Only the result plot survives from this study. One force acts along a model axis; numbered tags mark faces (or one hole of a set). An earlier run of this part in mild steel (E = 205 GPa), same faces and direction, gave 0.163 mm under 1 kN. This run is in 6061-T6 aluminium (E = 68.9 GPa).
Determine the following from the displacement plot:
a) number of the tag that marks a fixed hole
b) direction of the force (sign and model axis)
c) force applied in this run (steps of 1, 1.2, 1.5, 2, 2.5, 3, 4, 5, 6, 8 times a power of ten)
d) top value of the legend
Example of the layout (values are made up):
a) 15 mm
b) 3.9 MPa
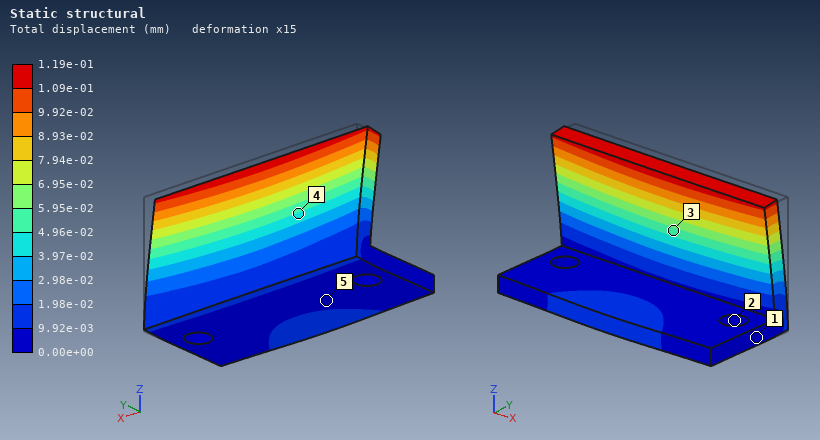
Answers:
a) 2
b) -Y
c) 250 N
d) 1.19e-01 mm
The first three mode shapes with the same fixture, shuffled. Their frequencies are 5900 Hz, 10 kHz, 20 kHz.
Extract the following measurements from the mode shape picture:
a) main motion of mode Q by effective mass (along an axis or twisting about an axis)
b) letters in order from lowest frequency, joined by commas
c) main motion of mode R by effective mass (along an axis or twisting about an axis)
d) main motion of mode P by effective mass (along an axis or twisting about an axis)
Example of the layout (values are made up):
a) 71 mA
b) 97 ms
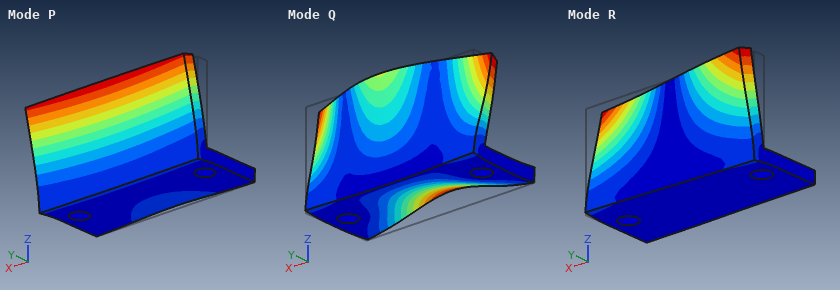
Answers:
a) along Z
b) P, R, Q
c) twisting about Z
d) along Y
